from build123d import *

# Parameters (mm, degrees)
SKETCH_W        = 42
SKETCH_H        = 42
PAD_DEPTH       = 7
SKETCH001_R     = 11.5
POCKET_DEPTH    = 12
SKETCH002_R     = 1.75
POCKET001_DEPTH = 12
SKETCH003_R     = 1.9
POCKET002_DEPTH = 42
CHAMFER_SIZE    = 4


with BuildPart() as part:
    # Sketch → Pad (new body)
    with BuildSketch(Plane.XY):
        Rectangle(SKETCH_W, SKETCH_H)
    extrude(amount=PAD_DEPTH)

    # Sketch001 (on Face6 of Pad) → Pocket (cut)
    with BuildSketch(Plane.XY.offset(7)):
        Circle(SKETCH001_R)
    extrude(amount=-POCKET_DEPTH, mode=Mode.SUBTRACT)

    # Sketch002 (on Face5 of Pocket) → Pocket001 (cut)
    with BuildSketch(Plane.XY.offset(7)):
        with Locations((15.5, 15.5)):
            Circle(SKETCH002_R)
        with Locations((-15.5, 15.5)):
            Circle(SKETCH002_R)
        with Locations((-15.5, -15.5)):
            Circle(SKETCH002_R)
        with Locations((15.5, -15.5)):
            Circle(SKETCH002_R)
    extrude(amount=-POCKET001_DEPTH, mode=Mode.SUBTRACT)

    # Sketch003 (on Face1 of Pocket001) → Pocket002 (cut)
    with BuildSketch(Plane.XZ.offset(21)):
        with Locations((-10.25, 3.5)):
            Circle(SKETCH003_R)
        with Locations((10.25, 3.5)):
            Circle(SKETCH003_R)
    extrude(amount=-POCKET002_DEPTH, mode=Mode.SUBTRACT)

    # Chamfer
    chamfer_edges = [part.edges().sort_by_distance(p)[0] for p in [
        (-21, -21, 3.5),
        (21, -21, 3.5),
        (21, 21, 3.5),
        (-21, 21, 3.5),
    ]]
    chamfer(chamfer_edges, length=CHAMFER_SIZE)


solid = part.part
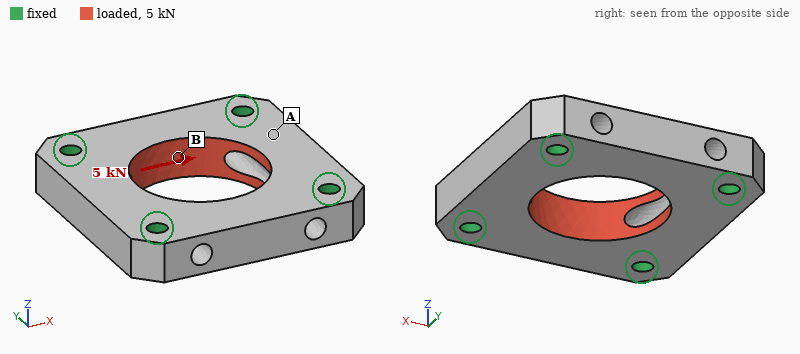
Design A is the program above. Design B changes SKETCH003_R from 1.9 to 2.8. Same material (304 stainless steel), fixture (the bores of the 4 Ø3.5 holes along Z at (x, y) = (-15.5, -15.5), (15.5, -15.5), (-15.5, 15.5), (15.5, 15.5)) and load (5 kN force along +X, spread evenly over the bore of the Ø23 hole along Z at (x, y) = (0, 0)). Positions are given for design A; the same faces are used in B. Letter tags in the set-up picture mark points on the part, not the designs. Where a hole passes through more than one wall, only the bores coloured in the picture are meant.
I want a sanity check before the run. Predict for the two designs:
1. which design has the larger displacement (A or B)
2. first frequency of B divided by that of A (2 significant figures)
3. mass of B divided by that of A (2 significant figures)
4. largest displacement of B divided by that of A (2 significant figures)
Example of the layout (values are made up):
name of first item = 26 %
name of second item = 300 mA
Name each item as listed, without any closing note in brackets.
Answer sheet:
which design has the larger displacement = B
first frequency of B divided by that of A = 0.60
mass of B divided by that of A = 0.89
largest displacement of B divided by that of A = 1.8
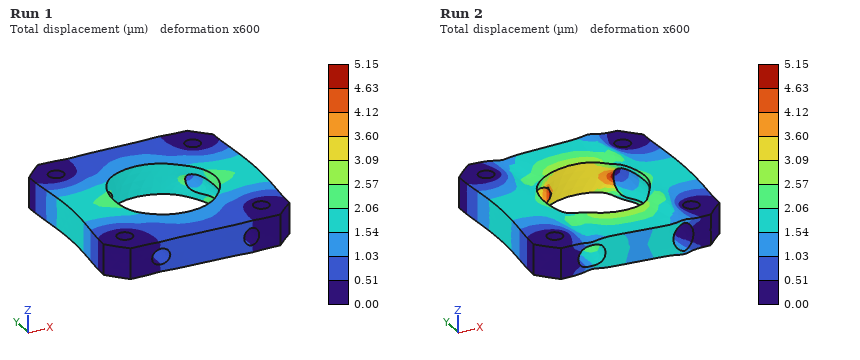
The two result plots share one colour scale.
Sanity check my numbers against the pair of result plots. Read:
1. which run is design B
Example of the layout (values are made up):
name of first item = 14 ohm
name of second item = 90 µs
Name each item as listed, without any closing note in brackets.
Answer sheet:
which run is design B = Run 2
